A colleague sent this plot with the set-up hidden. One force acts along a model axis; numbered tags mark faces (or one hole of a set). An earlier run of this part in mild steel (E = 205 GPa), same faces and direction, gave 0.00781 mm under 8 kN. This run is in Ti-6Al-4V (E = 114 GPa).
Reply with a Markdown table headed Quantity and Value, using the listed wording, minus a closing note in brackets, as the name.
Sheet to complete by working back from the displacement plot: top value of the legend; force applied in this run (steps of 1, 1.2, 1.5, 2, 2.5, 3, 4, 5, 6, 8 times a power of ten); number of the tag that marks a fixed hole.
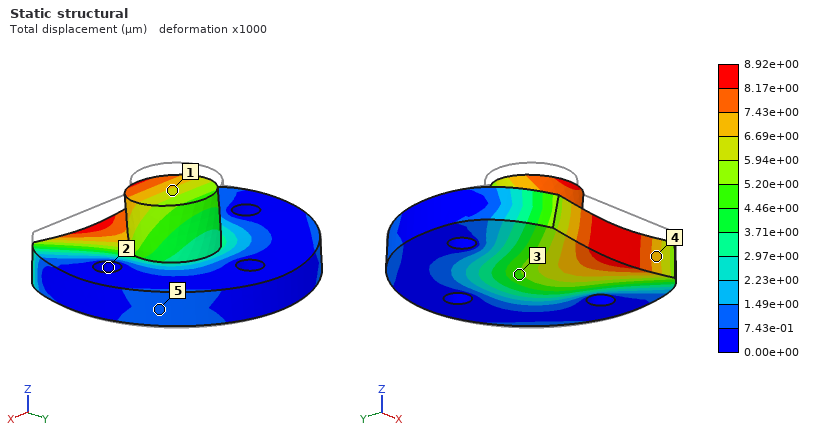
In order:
| Quantity | Value |
|---|---|
| top value of the legend | 8.92e+00 µm |
| force applied in this run | 5 kN |
| number of the tag that marks a fixed hole | 2 |
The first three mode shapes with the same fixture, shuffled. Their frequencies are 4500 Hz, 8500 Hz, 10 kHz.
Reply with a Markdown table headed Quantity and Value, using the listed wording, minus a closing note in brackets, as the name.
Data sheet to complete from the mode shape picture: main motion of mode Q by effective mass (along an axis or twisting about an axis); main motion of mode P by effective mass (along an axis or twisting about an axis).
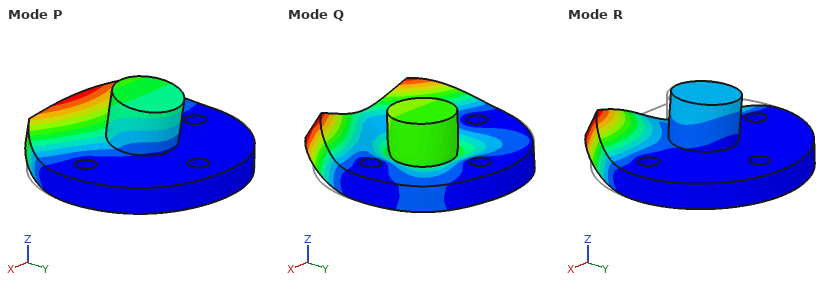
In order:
| Quantity | Value |
|---|---|
| main motion of mode Q by effective mass | along Z |
| main motion of mode P by effective mass | along Z |
